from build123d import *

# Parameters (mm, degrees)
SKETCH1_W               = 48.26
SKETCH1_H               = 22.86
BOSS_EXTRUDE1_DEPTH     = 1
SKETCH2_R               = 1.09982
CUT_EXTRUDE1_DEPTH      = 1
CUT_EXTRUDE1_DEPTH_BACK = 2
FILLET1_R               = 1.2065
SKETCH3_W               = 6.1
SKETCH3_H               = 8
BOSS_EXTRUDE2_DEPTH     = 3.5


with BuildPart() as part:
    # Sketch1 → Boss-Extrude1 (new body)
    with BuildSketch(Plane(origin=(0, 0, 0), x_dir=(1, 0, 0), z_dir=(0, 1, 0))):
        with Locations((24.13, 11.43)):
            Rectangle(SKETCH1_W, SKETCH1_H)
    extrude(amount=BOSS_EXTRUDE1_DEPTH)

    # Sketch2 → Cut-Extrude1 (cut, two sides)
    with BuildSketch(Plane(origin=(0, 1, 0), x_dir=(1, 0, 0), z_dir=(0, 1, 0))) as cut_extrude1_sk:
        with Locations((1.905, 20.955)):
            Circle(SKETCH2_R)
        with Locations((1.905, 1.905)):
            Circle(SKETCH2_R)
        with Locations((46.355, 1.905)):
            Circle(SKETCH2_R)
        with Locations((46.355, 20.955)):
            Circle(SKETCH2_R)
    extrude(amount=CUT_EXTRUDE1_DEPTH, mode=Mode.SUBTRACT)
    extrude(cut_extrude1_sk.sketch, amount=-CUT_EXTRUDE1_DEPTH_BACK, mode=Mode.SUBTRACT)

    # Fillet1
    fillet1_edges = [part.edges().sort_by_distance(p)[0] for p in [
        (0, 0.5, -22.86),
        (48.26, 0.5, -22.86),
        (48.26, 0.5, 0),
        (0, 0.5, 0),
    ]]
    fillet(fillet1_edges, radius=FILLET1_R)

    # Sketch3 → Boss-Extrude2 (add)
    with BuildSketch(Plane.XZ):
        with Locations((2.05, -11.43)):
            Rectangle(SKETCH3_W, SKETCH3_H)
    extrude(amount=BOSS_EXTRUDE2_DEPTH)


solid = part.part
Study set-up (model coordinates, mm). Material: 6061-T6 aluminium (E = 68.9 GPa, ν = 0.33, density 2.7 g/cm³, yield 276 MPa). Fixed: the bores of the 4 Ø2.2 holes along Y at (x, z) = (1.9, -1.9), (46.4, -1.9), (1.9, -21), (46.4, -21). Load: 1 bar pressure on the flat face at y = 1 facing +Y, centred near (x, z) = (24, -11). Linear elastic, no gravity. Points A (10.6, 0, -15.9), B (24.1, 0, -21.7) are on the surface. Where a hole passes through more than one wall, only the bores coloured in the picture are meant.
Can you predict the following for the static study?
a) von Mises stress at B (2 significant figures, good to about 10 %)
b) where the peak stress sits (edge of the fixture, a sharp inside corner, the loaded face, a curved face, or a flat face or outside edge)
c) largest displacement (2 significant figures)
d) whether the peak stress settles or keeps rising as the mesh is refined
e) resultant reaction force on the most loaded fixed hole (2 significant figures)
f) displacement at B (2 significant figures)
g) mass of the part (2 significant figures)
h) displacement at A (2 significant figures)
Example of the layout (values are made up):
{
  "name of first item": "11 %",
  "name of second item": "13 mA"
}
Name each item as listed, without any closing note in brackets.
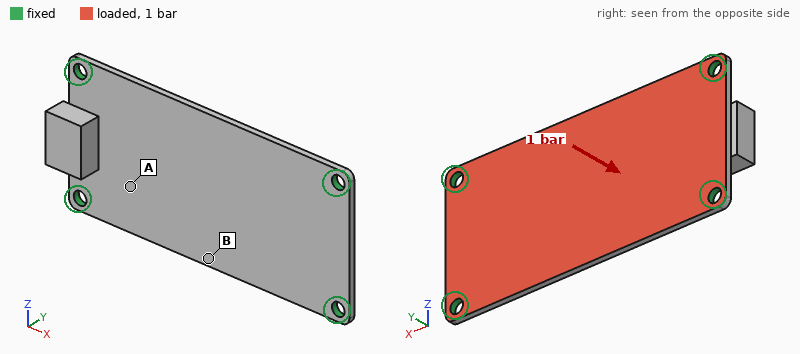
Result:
{
  "von Mises stress at B": "54 MPa",
  "where the peak stress sits": "edge of the fixture",
  "largest displacement": "0.20 mm",
  "whether the peak stress settles or keeps rising as the mesh is refined": "keeps rising",
  "resultant reaction force on the most loaded fixed hole": "28 N",
  "displacement at B": "0.19 mm",
  "mass of the part": "3.4 g",
  "displacement at A": "0.082 mm"
}
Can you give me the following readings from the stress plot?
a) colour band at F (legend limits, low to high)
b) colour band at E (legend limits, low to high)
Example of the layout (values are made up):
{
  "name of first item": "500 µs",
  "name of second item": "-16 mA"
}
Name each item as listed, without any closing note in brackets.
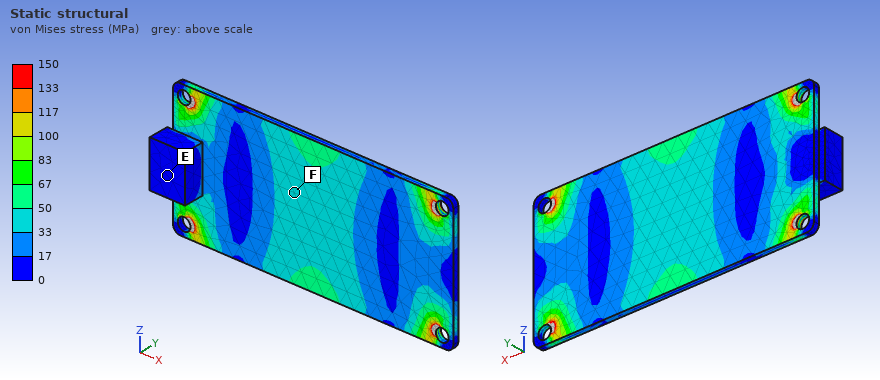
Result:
{
  "colour band at F": "33 to 50 MPa",
  "colour band at E": "0 to 17 MPa"
}
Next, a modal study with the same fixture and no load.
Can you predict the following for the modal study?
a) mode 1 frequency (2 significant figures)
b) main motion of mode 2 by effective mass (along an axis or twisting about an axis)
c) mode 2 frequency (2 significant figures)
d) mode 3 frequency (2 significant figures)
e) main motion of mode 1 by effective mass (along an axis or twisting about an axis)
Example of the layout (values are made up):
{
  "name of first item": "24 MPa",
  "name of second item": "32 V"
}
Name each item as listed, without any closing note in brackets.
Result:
{
  "mode 1 frequency": "2500 Hz",
  "main motion of mode 2 by effective mass": "twisting about X",
  "mode 2 frequency": "4500 Hz",
  "mode 3 frequency": "6900 Hz",
  "main motion of mode 1 by effective mass": "along Y"
}
